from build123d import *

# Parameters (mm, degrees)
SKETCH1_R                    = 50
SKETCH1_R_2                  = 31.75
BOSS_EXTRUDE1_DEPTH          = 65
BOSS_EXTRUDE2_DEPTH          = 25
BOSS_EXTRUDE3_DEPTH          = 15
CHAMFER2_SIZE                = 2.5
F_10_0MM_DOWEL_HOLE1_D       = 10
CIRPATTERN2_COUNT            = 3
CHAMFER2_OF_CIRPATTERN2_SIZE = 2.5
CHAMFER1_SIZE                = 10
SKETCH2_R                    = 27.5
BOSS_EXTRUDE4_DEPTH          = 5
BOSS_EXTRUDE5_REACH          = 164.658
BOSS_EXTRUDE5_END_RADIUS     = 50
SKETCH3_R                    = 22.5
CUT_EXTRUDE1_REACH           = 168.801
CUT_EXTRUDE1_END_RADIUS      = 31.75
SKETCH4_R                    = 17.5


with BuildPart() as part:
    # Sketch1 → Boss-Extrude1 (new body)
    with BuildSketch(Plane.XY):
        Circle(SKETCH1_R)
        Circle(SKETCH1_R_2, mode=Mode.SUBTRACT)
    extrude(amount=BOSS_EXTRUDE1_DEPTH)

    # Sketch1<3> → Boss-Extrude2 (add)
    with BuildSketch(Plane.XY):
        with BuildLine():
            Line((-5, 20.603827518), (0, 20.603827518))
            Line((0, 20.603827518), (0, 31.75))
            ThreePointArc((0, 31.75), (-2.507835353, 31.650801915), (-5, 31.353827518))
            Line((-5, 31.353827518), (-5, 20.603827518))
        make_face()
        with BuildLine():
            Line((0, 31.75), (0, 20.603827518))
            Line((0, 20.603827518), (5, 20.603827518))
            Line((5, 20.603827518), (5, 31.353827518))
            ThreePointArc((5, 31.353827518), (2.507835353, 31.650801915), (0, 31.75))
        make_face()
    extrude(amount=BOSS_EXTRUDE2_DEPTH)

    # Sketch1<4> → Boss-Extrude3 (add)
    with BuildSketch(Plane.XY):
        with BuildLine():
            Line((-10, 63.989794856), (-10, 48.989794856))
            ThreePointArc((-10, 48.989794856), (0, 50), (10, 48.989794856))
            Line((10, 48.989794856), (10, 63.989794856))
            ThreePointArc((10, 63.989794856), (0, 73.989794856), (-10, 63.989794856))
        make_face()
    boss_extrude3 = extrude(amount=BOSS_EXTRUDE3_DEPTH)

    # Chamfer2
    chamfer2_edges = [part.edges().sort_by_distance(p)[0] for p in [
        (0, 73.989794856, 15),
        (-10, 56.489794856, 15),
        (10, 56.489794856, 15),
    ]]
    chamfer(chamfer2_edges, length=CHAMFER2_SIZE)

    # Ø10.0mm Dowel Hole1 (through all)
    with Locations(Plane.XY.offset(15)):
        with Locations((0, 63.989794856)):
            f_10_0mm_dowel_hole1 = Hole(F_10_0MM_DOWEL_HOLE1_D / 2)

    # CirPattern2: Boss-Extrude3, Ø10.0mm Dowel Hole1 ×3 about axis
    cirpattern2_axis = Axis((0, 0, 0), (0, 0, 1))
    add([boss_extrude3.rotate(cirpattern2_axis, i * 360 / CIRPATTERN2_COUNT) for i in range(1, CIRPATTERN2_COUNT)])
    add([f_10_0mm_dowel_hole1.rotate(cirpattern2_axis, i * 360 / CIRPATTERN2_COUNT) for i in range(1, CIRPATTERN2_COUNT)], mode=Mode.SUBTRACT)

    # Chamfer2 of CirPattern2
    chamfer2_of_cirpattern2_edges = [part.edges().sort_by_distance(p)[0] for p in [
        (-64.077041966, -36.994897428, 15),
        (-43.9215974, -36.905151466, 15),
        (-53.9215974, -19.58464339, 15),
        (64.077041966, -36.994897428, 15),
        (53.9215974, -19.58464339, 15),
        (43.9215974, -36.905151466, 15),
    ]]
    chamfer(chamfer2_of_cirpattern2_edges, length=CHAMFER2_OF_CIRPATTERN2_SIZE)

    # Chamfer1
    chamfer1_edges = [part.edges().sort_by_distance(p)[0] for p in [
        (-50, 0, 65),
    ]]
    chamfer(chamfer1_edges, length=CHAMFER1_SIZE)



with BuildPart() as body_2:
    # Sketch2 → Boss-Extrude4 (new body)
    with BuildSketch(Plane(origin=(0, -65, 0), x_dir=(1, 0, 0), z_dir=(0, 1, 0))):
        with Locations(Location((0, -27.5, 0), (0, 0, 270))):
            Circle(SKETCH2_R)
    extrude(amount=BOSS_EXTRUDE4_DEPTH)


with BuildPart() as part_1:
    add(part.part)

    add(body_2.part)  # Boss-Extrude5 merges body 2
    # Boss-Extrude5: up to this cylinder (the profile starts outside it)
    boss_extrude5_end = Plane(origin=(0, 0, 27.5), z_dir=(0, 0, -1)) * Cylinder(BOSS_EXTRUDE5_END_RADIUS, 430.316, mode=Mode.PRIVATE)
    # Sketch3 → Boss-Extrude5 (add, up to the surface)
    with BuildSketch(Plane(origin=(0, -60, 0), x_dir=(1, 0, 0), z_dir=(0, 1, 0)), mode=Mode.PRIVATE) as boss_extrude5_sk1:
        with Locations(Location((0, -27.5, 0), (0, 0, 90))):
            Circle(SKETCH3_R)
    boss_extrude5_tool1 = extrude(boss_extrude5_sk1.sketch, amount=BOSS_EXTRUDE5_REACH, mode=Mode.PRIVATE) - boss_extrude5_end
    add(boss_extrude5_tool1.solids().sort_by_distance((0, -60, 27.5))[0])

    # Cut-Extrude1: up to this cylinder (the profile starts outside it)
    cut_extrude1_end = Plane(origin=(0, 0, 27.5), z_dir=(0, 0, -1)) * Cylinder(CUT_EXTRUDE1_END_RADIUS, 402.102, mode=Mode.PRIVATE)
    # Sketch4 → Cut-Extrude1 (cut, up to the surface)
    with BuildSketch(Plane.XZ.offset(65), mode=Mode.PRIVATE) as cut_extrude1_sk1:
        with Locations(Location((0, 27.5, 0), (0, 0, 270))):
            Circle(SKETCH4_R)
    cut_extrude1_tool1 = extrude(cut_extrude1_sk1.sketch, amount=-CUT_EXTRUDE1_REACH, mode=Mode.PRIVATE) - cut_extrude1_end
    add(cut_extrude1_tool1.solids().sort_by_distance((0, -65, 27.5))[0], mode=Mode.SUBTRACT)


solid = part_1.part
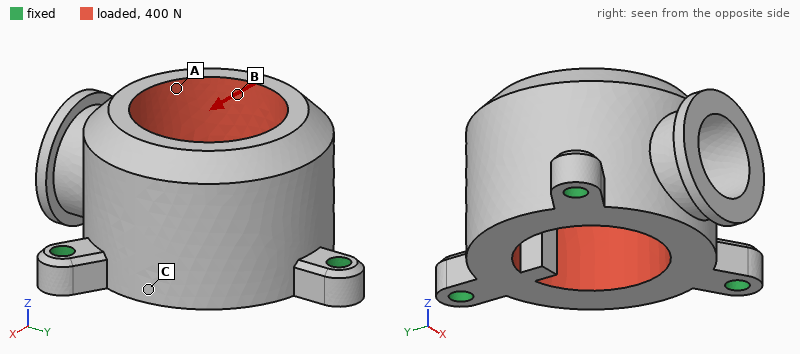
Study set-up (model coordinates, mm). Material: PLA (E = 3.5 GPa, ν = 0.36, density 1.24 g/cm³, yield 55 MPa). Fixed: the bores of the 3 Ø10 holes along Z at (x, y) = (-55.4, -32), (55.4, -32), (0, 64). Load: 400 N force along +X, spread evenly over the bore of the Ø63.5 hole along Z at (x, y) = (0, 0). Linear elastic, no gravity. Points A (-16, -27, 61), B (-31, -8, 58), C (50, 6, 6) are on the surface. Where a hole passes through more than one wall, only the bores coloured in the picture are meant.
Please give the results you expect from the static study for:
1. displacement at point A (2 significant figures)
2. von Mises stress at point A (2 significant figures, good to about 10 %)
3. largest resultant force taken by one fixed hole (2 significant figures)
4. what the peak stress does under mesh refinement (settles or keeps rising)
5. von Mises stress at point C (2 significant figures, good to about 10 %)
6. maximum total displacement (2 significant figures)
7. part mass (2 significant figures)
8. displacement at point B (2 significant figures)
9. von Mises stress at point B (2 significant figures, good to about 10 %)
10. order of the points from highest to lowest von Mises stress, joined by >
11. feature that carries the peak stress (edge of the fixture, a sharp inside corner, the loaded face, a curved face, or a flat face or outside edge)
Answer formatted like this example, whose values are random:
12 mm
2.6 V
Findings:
18 µm
0.54 MPa
180 N
keeps rising
0.14 MPa
27 µm
380 g
21 µm
0.27 MPa
A > B > C
edge of the fixture
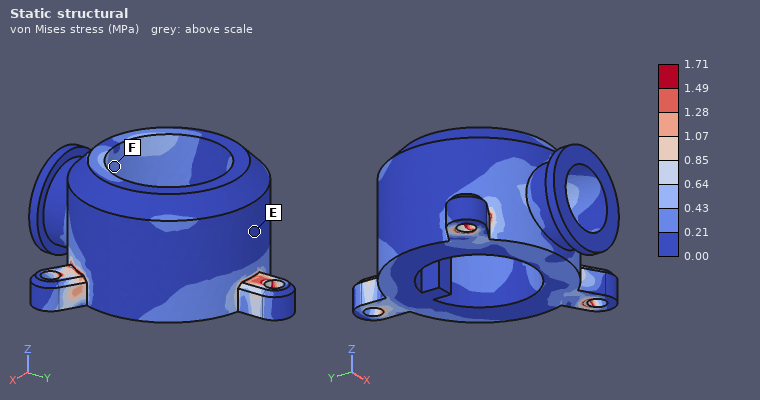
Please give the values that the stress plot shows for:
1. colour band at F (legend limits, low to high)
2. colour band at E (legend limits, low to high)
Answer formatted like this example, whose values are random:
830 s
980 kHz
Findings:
0.21 to 0.43 MPa
0.00 to 0.21 MPa
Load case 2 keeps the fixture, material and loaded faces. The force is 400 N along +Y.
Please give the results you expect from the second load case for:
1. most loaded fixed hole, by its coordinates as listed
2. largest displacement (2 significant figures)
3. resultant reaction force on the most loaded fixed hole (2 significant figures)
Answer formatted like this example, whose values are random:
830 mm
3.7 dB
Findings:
(0, 64)
26 µm
200 N
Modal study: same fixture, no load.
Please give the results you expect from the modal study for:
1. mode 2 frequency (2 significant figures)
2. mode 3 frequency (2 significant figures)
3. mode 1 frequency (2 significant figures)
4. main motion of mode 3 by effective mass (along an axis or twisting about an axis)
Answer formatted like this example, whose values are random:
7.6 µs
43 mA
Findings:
1200 Hz
1600 Hz
1200 Hz
along Z
